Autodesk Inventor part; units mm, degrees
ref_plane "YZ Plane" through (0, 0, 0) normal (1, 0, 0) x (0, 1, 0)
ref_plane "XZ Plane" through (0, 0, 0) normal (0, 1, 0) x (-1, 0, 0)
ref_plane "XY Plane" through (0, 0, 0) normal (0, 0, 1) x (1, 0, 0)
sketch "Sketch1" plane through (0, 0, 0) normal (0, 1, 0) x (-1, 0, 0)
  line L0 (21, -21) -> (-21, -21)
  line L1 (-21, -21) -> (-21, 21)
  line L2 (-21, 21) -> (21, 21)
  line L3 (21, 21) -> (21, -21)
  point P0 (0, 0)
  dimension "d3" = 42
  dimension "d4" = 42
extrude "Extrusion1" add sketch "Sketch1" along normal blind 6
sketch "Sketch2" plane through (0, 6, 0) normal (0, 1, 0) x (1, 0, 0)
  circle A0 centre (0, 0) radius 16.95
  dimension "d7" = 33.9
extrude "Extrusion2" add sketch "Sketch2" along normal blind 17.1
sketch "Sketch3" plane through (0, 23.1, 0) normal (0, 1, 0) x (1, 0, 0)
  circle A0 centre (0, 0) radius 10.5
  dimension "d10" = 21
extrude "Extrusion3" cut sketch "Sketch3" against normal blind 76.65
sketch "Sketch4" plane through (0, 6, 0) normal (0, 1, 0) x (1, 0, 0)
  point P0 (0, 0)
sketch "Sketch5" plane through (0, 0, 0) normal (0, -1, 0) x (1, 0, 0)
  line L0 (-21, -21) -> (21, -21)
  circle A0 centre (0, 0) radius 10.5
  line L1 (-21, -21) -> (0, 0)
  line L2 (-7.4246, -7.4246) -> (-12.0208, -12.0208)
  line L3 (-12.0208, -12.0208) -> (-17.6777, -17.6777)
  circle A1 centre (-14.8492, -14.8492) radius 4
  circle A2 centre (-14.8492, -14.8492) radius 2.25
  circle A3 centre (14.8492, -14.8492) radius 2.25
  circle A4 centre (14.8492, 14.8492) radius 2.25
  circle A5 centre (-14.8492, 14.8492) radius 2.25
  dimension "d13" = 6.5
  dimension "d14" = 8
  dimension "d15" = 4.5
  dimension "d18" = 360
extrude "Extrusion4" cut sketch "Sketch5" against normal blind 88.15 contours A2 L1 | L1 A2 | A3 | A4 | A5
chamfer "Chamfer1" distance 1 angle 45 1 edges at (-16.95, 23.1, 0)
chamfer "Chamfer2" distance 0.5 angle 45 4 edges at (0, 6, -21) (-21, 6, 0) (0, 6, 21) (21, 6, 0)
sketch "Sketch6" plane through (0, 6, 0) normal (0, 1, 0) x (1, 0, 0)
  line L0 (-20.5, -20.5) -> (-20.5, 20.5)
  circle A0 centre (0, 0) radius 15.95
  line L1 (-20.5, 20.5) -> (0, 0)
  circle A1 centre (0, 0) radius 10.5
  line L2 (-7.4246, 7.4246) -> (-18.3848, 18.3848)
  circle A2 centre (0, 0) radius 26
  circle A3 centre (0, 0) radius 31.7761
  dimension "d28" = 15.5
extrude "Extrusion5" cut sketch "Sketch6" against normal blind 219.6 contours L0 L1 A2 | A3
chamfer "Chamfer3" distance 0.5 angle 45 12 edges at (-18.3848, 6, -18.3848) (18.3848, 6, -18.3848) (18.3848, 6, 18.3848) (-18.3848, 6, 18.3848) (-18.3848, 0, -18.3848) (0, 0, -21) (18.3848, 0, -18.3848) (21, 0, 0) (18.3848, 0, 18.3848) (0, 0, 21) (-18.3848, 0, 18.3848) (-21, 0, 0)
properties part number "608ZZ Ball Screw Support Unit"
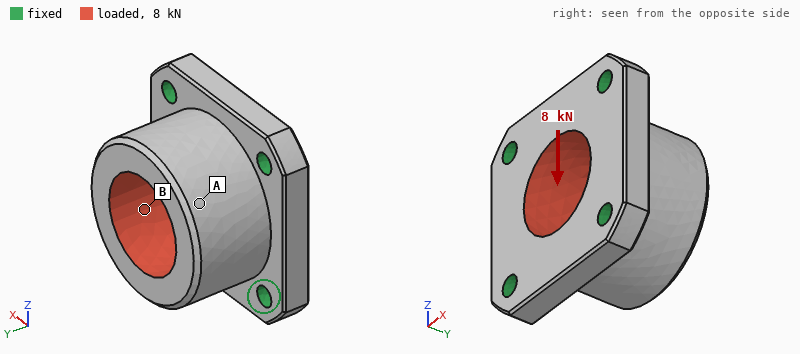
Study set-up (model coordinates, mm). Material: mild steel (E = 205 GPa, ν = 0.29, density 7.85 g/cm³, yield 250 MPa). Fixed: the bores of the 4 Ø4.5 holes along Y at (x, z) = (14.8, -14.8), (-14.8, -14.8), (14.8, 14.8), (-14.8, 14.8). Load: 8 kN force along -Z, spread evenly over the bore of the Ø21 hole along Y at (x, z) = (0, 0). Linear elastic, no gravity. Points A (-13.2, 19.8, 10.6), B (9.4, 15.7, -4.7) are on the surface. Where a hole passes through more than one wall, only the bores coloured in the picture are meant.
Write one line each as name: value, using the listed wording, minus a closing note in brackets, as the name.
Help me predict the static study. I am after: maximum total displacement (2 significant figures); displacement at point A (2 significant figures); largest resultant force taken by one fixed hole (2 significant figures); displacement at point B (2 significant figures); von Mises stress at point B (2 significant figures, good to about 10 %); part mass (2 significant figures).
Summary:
maximum total displacement: 6.9 µm
displacement at point A: 5.2 µm
largest resultant force taken by one fixed hole: 2.4 kN
displacement at point B: 4.2 µm
von Mises stress at point B: 25 MPa
part mass: 140 g
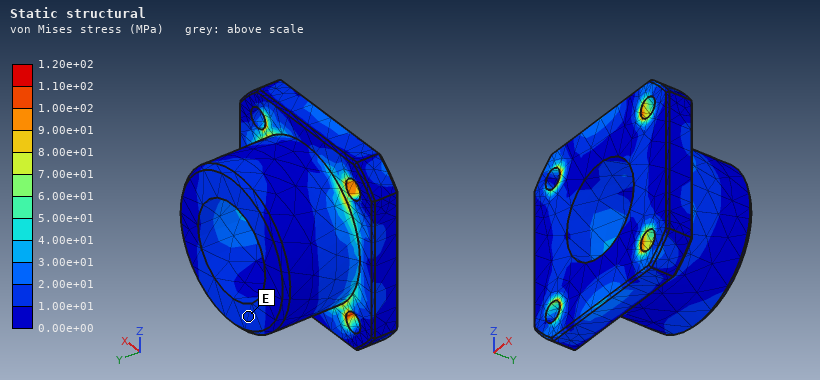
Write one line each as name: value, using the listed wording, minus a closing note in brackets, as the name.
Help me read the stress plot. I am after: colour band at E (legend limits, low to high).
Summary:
colour band at E: 1.00e+01 to 2.00e+01 MPa
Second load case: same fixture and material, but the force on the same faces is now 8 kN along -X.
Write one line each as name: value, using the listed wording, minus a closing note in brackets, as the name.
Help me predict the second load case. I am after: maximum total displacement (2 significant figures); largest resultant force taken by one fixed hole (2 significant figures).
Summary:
maximum total displacement: 6.9 µm
largest resultant force taken by one fixed hole: 2.4 kN
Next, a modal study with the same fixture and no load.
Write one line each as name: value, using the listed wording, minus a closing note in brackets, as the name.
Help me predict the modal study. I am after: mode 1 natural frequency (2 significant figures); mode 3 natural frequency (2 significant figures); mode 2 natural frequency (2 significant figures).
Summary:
mode 1 natural frequency: 20 kHz
mode 3 natural frequency: 24 kHz
mode 2 natural frequency: 20 kHz
